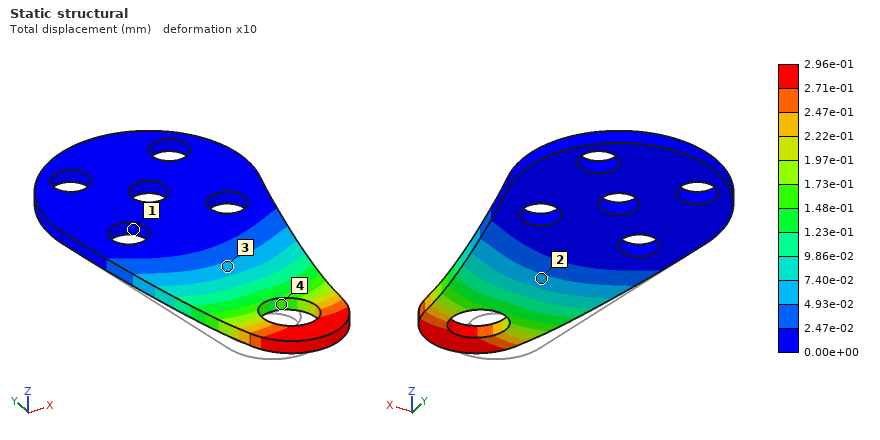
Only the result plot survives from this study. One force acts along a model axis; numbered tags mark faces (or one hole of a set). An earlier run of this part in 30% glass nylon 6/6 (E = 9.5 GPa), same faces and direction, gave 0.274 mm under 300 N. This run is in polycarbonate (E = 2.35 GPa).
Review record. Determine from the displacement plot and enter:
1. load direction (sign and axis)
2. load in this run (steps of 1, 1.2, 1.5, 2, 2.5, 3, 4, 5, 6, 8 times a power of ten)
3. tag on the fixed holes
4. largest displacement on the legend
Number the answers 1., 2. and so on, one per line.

1. +X
2. 80 N
3. 1
4. 2.96e-01 mm
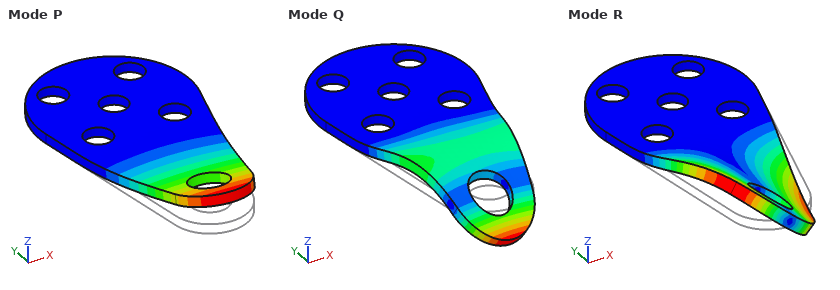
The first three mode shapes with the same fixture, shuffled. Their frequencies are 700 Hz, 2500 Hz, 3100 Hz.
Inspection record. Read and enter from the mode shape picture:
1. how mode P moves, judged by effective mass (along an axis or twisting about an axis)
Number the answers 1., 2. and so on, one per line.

1. along Z
